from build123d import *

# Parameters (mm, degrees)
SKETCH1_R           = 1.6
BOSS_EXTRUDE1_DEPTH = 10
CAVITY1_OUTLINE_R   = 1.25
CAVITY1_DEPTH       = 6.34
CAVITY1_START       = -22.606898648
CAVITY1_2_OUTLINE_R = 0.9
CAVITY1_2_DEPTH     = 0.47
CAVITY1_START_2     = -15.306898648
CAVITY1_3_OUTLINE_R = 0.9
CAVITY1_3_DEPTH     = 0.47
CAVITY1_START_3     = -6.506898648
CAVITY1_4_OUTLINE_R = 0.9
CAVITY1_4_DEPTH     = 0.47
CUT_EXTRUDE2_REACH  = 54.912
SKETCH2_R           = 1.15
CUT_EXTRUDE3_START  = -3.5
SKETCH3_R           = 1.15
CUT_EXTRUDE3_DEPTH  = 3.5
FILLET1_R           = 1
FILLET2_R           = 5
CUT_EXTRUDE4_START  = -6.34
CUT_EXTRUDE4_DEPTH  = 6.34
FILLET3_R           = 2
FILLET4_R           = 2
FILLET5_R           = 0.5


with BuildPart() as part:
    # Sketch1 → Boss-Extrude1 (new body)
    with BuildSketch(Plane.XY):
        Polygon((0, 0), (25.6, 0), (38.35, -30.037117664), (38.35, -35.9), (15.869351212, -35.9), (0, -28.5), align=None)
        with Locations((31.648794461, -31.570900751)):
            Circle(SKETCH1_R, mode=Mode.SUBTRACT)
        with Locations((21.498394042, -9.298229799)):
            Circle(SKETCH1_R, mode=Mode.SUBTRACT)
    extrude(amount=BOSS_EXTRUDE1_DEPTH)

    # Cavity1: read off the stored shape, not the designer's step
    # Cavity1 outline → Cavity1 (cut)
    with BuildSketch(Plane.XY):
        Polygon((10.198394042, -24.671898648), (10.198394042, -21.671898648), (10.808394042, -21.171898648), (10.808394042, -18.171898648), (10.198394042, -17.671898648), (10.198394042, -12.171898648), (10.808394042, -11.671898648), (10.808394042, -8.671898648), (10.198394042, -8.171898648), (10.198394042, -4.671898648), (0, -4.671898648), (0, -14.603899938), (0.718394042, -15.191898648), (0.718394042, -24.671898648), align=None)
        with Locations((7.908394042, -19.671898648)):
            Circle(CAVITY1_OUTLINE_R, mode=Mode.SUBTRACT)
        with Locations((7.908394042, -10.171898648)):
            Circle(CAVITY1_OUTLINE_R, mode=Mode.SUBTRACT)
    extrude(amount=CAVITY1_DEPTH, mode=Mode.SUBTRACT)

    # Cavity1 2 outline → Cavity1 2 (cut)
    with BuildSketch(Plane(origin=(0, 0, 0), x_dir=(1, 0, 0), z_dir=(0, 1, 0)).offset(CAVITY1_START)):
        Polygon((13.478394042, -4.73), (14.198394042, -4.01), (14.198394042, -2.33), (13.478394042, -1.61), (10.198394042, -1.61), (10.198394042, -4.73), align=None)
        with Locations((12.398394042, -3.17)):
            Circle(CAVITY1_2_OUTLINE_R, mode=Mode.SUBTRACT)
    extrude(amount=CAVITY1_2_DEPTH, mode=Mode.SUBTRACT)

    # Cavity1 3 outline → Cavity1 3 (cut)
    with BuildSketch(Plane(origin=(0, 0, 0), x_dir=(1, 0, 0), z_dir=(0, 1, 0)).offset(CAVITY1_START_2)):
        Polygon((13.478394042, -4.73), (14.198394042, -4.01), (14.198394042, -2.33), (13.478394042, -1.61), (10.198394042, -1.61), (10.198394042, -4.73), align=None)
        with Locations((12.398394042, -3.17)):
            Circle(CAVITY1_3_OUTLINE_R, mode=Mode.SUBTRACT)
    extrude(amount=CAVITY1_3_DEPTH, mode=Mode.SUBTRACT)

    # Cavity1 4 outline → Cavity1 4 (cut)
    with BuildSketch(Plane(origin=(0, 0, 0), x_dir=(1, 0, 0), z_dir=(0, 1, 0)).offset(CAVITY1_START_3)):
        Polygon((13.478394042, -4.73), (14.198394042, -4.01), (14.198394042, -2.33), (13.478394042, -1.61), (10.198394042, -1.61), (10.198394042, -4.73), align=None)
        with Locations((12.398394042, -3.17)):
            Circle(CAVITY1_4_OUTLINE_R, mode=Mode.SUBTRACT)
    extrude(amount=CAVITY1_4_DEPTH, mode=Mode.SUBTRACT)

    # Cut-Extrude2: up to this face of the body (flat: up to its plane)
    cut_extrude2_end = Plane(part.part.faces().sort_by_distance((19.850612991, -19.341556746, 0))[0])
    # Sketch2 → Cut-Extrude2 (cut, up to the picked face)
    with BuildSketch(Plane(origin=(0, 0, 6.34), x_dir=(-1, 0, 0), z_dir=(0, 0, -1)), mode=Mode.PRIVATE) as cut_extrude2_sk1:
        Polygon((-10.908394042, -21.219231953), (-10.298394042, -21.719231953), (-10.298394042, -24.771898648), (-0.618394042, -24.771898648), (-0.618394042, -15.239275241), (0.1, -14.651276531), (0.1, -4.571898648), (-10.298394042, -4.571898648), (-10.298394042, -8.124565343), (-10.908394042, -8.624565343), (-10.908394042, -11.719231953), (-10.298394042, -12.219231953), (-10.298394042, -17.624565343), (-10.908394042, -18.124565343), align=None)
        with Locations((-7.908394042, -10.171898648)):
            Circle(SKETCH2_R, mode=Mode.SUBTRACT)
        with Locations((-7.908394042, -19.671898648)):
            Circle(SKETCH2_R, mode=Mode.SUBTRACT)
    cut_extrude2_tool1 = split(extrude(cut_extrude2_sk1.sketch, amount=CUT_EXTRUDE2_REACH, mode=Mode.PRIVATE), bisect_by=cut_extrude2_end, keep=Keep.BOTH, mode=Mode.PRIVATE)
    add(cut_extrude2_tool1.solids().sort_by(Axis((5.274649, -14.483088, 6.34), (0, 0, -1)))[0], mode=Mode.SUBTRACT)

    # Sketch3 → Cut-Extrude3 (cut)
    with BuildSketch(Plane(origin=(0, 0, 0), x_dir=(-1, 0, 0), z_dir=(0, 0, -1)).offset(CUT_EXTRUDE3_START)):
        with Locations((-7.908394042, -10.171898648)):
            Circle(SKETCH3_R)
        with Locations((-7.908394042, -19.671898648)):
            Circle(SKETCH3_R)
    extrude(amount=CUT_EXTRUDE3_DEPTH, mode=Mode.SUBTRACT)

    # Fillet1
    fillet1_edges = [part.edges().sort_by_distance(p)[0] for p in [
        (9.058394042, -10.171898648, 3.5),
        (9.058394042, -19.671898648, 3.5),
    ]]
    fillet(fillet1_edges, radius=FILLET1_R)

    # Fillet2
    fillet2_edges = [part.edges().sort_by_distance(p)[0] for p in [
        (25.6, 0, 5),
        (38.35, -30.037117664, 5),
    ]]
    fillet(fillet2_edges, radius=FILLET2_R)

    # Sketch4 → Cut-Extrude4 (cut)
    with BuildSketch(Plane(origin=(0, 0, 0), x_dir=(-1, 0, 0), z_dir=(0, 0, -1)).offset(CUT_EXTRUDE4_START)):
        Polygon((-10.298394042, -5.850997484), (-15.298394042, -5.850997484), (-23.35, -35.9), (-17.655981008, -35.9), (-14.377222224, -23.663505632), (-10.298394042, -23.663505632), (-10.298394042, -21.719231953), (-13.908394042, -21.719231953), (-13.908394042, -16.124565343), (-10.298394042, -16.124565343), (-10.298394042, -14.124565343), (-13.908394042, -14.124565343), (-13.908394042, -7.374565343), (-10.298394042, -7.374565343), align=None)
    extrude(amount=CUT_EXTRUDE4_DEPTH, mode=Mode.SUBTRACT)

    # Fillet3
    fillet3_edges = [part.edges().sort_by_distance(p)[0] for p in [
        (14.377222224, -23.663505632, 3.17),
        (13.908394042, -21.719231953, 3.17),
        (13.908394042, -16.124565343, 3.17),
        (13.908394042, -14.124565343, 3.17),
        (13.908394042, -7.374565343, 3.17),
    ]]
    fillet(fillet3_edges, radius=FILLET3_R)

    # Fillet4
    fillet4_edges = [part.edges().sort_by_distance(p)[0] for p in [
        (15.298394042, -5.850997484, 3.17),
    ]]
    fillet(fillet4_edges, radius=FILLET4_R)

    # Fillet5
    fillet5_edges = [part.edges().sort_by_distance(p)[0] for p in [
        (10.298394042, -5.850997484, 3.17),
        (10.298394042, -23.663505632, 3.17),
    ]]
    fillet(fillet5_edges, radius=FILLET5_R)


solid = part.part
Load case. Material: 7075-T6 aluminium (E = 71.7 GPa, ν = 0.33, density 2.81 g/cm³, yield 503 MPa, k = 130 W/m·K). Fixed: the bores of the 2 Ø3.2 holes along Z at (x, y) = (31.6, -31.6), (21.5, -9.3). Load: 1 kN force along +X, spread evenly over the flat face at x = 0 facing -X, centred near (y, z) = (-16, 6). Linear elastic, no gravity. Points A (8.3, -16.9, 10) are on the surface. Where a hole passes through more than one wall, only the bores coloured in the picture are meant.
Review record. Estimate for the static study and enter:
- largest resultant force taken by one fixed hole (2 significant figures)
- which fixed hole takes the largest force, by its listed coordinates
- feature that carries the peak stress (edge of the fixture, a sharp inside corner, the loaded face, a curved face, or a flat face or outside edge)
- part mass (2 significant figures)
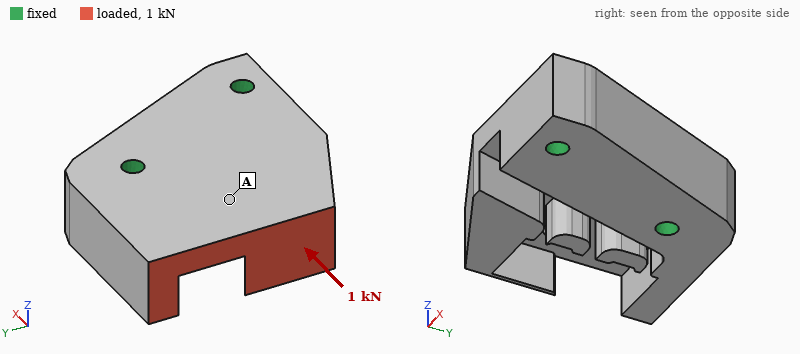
670 N
(21.5, -9.3)
the loaded face
25 g
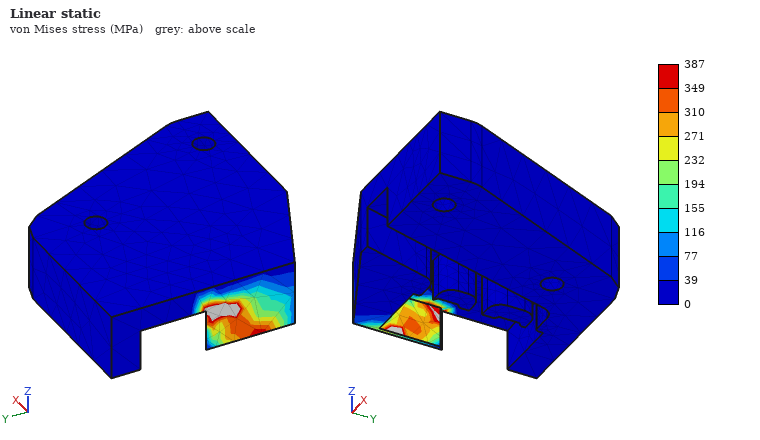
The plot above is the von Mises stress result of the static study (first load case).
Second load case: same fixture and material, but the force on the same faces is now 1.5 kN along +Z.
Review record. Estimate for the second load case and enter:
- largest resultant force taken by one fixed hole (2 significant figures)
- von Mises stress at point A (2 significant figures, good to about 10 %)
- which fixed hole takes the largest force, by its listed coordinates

1.4 kN
92 MPa
(21.5, -9.3)
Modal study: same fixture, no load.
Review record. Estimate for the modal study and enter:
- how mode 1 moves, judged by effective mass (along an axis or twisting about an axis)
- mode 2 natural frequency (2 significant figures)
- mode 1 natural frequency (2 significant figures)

along Z
14 kHz
6600 Hz
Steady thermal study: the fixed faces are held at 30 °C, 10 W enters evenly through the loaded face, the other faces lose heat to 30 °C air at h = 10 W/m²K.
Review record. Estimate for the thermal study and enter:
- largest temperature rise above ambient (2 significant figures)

23 K
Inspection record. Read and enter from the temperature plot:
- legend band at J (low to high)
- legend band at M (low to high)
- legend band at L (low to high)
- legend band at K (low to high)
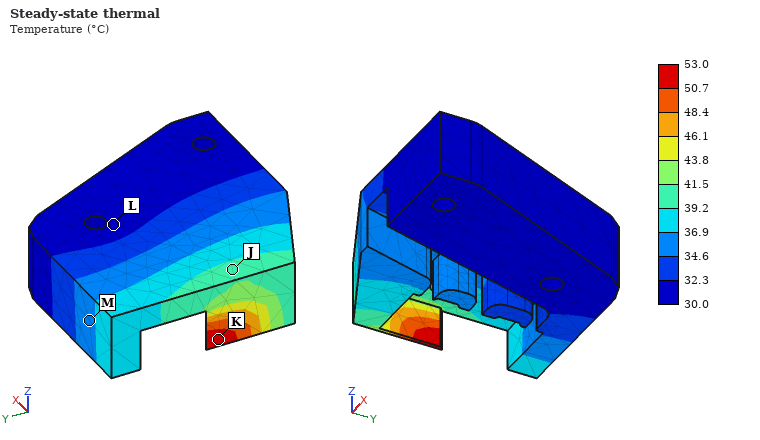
39.2 to 41.5 °C
34.6 to 36.9 °C
30.0 to 32.3 °C
50.7 to 53.0 °C
